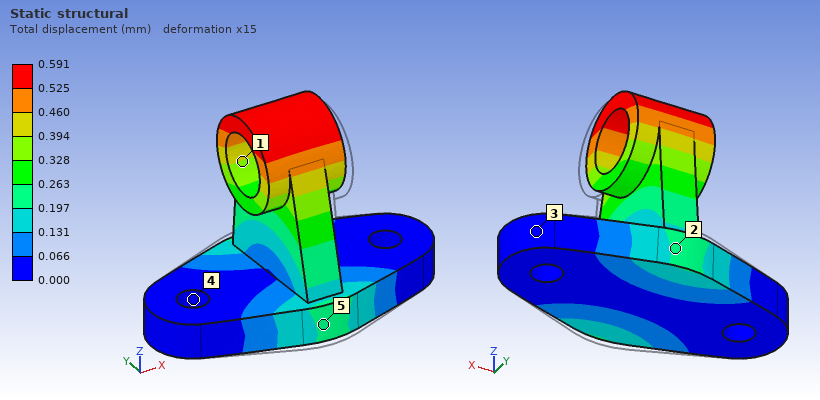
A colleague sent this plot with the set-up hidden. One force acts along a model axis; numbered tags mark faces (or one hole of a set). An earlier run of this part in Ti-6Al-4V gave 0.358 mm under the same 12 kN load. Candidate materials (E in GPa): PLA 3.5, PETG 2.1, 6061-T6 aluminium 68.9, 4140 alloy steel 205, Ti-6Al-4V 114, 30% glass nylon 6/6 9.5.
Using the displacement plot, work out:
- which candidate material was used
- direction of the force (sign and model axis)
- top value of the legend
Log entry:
6061-T6 aluminium
+Y
0.591 mm
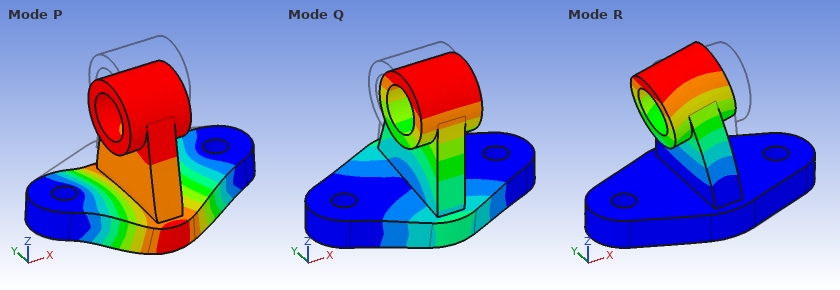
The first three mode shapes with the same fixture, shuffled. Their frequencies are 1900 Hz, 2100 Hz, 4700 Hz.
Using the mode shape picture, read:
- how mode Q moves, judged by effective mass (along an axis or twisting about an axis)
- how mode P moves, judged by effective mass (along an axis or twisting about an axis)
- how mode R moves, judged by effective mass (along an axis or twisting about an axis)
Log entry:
along Y
along Z
along X
